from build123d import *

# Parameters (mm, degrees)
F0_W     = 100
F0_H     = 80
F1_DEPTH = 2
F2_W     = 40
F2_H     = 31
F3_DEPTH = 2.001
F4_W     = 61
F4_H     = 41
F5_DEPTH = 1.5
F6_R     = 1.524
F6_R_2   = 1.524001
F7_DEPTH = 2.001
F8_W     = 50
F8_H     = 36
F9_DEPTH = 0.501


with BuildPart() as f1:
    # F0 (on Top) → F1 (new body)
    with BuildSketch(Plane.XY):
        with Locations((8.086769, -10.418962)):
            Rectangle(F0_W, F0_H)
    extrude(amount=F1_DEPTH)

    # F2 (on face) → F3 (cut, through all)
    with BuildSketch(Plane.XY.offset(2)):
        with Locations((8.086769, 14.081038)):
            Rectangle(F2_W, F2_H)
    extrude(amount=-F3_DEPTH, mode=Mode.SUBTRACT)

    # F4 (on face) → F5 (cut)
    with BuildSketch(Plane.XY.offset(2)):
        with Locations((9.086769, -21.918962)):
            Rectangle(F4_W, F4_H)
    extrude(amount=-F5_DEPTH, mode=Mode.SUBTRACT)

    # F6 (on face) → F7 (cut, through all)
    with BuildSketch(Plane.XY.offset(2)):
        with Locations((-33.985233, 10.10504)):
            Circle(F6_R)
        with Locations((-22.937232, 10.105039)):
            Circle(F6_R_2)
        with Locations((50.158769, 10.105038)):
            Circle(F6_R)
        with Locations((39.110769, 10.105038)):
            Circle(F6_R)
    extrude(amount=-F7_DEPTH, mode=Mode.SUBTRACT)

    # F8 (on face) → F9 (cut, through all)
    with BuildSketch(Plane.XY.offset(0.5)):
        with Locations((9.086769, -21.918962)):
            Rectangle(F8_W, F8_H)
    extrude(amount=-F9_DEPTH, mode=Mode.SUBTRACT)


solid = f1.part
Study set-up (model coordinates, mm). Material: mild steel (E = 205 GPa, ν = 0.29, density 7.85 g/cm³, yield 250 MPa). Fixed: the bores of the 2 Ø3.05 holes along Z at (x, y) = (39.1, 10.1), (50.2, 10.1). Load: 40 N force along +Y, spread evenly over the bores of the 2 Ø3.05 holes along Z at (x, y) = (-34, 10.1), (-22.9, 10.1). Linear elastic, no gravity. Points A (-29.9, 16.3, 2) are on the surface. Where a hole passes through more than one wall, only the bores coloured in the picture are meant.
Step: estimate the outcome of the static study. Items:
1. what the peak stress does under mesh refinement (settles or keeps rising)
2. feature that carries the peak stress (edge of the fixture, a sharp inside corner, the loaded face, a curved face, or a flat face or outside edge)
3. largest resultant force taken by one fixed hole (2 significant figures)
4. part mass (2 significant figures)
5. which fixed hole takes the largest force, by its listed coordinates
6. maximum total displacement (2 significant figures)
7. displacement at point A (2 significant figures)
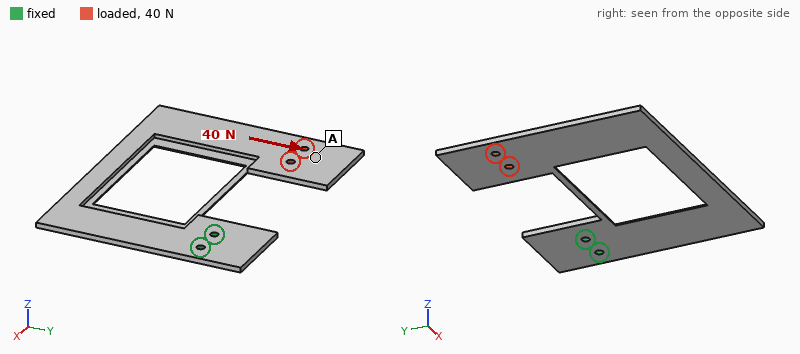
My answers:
keeps rising
a sharp inside corner
250 N
69 g
(39.1, 10.1)
0.19 mm
0.088 mm
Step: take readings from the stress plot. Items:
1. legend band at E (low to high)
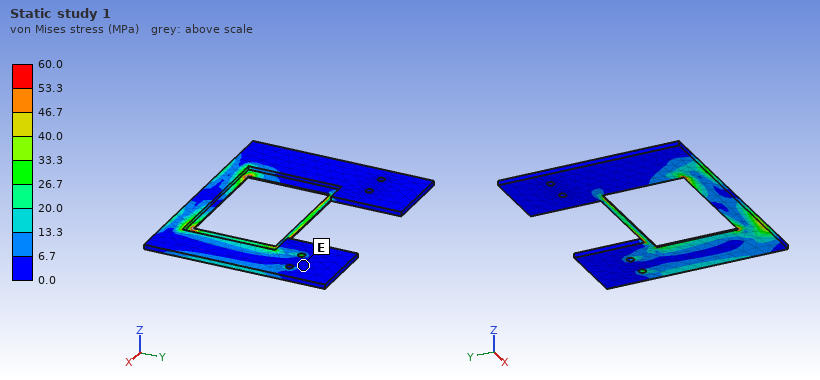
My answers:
0.0 to 6.7 MPa
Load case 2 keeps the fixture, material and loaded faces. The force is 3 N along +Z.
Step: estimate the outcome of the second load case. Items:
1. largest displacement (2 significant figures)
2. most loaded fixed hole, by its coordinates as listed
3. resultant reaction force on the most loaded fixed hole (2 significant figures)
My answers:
1.3 mm
(39.1, 10.1)
15 N
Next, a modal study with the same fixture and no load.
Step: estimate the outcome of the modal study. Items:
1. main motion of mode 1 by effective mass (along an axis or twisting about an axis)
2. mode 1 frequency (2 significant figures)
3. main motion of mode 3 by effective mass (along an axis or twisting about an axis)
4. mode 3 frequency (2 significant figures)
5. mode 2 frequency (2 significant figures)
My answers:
along Z
57 Hz
along Z
420 Hz
140 Hz
